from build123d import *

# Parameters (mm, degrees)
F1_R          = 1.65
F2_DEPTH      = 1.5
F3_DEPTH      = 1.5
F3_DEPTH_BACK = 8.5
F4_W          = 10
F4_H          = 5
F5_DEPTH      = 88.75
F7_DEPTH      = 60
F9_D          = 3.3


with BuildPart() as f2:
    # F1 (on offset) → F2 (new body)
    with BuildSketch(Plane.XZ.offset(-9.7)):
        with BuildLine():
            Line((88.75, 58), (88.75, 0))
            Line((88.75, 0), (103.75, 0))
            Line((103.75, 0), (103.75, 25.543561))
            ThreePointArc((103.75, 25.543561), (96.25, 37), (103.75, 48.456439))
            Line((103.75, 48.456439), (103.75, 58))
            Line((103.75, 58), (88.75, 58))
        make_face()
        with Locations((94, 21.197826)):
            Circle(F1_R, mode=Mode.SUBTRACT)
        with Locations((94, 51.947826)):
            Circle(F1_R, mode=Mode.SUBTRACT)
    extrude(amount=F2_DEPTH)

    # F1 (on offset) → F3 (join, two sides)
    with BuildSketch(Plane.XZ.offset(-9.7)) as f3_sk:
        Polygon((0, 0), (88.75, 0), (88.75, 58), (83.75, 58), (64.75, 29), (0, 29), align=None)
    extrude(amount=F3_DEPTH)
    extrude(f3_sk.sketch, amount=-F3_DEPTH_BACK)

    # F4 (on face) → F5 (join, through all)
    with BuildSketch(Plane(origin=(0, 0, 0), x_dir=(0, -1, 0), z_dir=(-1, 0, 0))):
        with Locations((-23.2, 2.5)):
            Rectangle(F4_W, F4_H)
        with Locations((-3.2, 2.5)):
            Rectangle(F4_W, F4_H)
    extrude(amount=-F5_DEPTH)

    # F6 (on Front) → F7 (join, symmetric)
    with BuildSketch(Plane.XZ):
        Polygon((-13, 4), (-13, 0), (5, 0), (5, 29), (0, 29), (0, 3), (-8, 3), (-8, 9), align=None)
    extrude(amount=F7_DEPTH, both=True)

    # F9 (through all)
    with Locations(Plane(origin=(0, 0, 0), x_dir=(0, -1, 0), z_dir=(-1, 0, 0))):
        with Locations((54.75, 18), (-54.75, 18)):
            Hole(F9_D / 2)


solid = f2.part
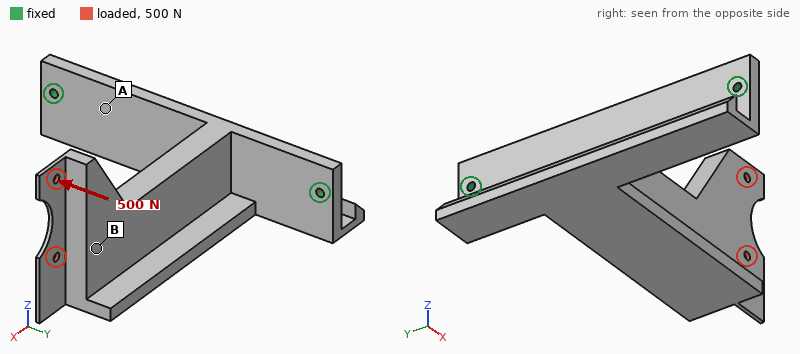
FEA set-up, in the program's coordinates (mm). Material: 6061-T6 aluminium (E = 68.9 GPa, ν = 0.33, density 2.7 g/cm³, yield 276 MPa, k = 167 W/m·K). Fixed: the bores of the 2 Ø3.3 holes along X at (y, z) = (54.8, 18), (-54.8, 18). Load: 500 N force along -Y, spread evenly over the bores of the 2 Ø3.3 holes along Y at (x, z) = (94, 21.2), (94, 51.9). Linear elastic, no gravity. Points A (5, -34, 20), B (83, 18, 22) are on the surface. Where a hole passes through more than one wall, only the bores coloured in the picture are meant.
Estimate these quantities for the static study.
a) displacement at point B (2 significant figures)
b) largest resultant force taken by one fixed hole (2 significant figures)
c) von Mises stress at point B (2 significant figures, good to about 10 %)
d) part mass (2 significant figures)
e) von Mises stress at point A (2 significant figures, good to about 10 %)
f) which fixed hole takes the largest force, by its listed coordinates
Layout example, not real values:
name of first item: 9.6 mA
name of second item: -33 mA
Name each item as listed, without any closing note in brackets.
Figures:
displacement at point B: 0.41 mm
largest resultant force taken by one fixed hole: 650 N
von Mises stress at point B: 23 MPa
part mass: 170 g
von Mises stress at point A: 12 MPa
which fixed hole takes the largest force, by its listed coordinates: (54.8, 18)
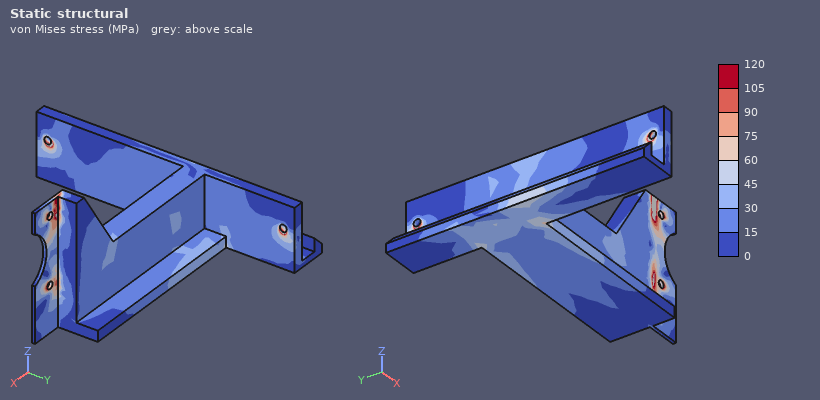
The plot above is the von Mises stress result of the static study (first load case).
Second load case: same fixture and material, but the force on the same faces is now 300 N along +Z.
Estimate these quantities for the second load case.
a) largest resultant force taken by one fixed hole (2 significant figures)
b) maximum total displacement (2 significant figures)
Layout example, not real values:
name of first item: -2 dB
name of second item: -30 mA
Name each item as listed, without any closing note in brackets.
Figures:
largest resultant force taken by one fixed hole: 380 N
maximum total displacement: 1.9 mm
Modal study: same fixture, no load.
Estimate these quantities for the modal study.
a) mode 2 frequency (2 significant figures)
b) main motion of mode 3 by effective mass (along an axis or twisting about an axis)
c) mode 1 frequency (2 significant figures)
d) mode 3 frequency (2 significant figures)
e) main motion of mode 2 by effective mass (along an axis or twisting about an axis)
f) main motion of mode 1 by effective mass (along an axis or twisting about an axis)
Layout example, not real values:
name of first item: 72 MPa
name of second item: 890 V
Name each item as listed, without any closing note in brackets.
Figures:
mode 2 frequency: 910 Hz
main motion of mode 3 by effective mass: along X
mode 1 frequency: 340 Hz
mode 3 frequency: 1500 Hz
main motion of mode 2 by effective mass: along Y
main motion of mode 1 by effective mass: along Z
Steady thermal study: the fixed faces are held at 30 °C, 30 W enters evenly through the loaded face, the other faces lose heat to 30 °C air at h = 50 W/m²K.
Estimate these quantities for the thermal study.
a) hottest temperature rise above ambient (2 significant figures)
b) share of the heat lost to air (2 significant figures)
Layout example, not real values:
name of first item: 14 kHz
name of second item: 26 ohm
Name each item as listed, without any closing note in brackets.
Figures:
hottest temperature rise above ambient: 74 K
share of the heat lost to air: 66 %
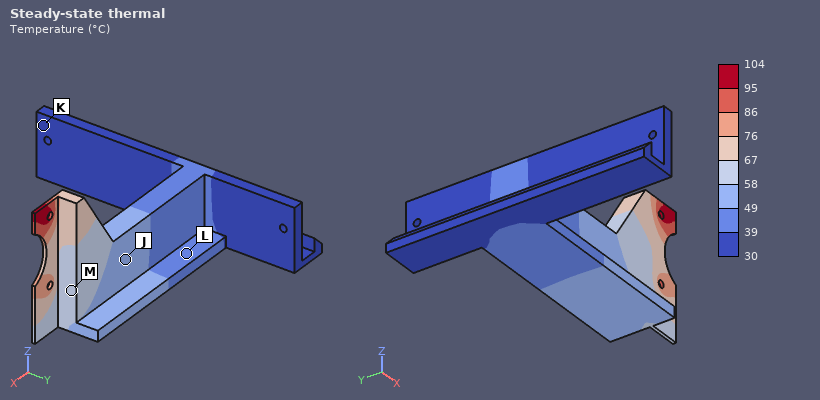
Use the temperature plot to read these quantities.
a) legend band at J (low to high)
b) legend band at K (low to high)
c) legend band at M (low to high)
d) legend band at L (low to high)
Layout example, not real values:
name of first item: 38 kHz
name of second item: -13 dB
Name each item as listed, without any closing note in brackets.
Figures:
legend band at J: 49 to 58 °C
legend band at K: 30 to 39 °C
legend band at M: 58 to 67 °C
legend band at L: 39 to 49 °C
